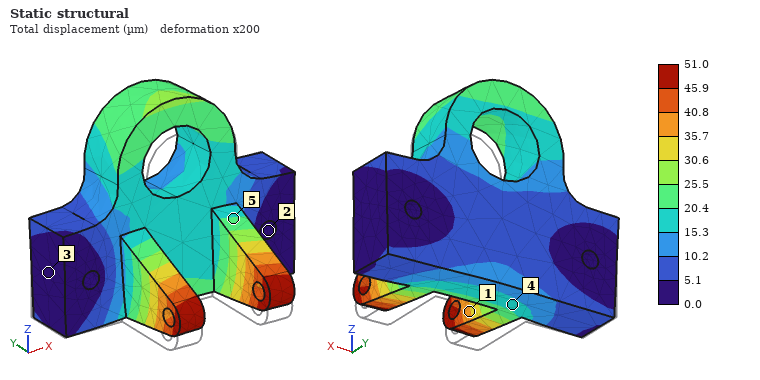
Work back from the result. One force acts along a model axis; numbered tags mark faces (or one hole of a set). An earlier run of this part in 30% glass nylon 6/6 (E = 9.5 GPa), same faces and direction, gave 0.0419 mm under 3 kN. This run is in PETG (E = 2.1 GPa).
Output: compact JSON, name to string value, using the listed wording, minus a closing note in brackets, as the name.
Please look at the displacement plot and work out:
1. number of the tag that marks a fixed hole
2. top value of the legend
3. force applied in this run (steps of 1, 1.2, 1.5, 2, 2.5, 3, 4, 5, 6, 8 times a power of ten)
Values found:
{"number of the tag that marks a fixed hole": "2", "top value of the legend": "51.0 µm", "force applied in this run": "800 N"}
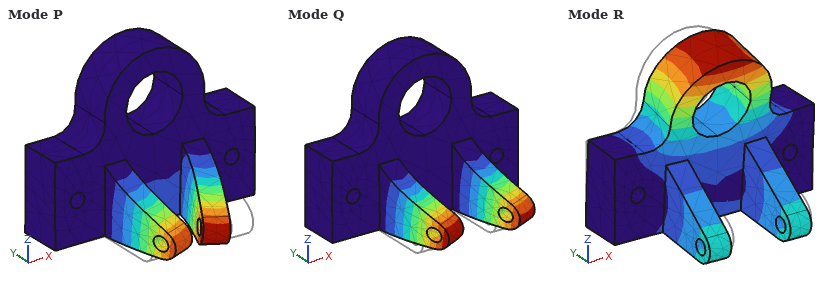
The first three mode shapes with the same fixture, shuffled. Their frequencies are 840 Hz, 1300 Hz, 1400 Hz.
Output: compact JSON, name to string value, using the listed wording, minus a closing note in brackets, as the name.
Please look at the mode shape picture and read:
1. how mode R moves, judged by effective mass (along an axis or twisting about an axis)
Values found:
{"how mode R moves, judged by effective mass": "along Y"}
